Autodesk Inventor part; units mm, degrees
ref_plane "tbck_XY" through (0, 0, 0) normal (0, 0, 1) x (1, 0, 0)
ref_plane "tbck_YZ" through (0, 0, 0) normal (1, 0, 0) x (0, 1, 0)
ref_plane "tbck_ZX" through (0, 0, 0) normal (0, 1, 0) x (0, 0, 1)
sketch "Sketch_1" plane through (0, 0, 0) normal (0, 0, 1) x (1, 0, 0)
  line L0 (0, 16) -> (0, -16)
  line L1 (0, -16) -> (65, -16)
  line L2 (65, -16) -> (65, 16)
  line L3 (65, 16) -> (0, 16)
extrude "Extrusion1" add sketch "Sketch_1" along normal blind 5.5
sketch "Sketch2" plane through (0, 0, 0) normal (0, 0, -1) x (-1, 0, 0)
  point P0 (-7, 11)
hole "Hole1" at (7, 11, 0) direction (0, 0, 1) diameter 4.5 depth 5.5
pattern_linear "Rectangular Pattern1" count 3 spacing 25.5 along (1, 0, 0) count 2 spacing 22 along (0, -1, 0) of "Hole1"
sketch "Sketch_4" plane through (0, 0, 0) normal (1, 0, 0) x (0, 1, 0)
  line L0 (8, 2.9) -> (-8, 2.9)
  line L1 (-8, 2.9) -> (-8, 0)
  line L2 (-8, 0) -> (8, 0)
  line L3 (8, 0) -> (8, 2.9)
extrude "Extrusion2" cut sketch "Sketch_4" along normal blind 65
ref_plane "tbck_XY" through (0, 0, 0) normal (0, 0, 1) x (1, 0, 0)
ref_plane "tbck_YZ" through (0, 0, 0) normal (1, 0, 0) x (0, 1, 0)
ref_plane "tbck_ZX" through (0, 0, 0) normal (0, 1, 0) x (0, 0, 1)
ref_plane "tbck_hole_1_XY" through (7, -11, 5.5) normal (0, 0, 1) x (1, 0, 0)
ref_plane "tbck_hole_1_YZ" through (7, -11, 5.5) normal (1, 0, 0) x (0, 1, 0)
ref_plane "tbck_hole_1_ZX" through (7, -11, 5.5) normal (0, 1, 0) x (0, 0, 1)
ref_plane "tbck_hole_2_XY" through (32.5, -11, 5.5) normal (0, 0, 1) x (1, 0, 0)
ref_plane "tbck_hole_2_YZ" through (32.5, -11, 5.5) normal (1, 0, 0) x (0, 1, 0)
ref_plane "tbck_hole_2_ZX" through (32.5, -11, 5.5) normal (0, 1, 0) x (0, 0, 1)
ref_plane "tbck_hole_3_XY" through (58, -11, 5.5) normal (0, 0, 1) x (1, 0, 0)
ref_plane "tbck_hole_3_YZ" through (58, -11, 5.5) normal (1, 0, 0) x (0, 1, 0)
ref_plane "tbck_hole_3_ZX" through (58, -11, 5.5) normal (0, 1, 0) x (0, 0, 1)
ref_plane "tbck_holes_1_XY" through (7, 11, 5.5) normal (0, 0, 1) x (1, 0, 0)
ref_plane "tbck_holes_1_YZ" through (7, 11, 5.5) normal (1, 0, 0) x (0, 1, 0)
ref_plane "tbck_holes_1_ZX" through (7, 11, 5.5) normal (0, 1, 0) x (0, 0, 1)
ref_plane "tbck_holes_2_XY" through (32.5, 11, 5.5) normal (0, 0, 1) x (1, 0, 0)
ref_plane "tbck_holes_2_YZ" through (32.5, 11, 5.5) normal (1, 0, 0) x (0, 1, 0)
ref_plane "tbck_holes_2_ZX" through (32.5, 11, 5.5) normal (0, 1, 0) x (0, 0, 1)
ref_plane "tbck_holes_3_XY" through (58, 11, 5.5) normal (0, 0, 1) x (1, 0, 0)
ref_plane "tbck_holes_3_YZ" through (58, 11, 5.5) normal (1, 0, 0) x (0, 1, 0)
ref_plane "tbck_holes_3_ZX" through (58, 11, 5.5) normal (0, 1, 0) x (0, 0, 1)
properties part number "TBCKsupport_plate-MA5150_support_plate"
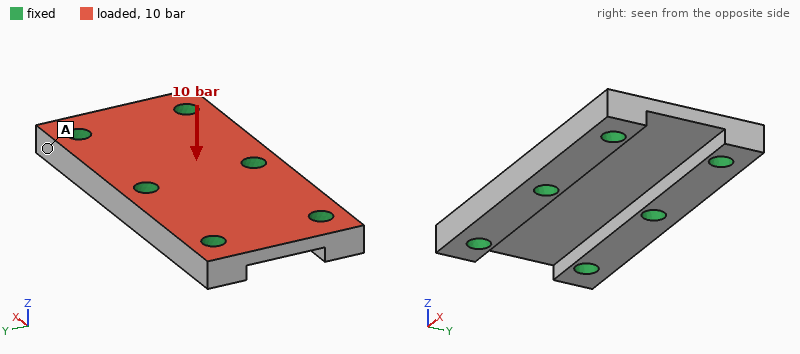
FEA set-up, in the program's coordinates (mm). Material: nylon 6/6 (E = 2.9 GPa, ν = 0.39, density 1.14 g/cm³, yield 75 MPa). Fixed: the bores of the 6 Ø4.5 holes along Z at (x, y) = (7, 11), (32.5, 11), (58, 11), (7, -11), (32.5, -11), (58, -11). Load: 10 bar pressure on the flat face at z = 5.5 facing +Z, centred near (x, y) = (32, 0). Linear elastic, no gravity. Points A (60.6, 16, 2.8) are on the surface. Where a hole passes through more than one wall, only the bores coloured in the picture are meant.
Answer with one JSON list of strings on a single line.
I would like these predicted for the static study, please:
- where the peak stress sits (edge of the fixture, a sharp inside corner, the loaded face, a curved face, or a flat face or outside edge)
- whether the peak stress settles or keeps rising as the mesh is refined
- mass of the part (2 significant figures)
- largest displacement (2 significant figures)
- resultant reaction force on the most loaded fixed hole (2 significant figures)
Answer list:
["edge of the fixture", "keeps rising", "9.0 g", "0.14 mm", "400 N"]
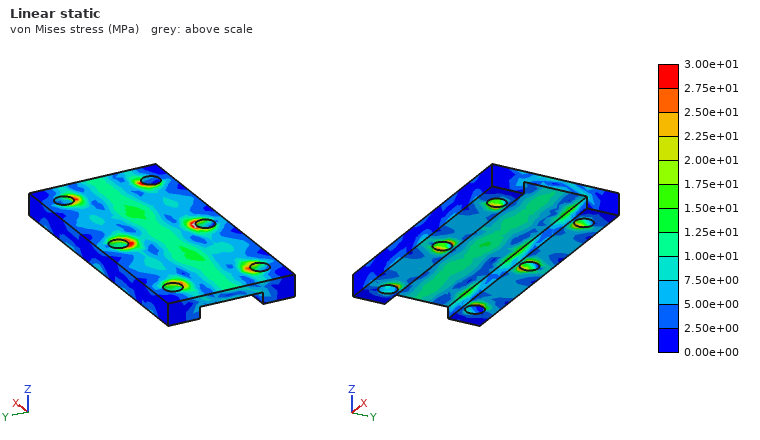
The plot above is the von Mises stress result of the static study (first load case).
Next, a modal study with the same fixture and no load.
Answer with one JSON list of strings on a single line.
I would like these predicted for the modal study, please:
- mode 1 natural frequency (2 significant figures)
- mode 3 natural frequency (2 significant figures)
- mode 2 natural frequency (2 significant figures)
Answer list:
["9300 Hz", "12 kHz", "9300 Hz"]
